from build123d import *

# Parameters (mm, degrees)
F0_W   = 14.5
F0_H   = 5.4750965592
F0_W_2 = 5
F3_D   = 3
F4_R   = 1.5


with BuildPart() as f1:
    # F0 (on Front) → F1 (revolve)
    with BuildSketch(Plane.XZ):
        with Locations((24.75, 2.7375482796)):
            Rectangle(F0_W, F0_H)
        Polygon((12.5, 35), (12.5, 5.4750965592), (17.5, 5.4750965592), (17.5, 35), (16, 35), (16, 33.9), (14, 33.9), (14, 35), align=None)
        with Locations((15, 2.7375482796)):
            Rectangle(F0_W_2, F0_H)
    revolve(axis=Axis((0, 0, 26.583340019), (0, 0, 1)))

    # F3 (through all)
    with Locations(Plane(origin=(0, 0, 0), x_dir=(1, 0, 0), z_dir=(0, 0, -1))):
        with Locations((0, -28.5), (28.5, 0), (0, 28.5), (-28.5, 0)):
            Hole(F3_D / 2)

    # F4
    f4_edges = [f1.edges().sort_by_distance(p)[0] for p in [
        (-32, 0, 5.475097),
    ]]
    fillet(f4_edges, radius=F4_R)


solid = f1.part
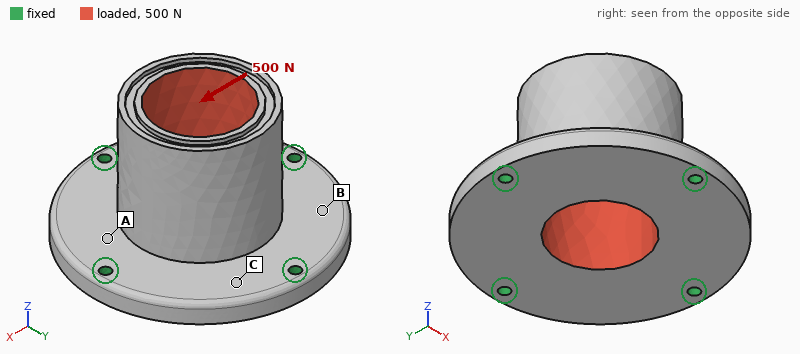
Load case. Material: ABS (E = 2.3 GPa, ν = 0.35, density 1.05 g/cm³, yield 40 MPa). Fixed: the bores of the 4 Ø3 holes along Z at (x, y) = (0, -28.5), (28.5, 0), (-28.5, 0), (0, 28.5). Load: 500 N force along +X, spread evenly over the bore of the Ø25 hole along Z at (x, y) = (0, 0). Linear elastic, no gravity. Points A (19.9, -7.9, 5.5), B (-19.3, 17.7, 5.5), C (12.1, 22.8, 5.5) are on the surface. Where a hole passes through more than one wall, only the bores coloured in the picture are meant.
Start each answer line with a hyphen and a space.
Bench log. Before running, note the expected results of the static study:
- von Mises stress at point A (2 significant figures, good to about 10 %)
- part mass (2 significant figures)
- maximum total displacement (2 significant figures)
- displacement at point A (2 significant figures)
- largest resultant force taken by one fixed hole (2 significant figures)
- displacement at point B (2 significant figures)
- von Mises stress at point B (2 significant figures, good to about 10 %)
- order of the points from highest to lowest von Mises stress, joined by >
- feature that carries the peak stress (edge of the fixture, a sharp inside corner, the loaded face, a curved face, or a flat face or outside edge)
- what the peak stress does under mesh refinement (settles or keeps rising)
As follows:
- 4.1 MPa
- 30 g
- 0.19 mm
- 0.047 mm
- 210 N
- 0.047 mm
- 1.9 MPa
- A > B > C
- edge of the fixture
- keeps rising
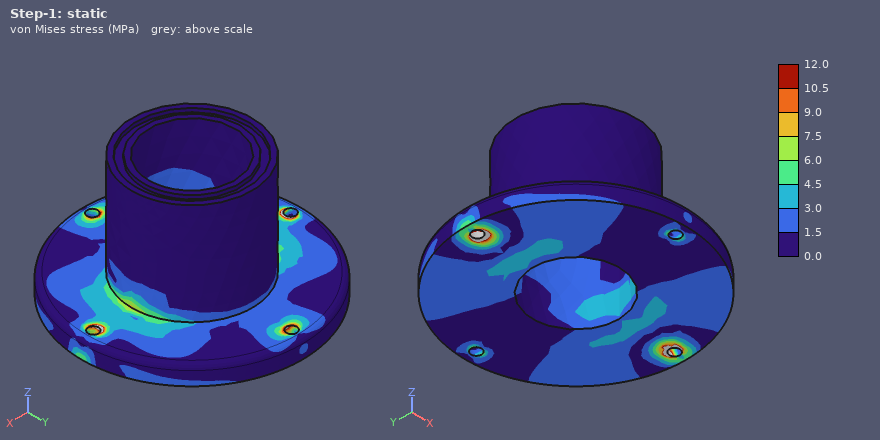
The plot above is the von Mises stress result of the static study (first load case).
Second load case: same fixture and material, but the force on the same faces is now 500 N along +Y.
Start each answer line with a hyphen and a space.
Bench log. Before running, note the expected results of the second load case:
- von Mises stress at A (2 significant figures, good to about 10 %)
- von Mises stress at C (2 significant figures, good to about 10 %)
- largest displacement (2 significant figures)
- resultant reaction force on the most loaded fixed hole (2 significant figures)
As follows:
- 1.4 MPa
- 2.4 MPa
- 0.19 mm
- 210 N
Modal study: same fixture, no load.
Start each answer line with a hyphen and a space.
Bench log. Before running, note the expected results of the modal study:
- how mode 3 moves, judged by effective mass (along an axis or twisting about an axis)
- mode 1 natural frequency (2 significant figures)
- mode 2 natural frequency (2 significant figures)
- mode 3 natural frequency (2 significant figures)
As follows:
- along Z
- 2200 Hz
- 2200 Hz
- 2600 Hz
